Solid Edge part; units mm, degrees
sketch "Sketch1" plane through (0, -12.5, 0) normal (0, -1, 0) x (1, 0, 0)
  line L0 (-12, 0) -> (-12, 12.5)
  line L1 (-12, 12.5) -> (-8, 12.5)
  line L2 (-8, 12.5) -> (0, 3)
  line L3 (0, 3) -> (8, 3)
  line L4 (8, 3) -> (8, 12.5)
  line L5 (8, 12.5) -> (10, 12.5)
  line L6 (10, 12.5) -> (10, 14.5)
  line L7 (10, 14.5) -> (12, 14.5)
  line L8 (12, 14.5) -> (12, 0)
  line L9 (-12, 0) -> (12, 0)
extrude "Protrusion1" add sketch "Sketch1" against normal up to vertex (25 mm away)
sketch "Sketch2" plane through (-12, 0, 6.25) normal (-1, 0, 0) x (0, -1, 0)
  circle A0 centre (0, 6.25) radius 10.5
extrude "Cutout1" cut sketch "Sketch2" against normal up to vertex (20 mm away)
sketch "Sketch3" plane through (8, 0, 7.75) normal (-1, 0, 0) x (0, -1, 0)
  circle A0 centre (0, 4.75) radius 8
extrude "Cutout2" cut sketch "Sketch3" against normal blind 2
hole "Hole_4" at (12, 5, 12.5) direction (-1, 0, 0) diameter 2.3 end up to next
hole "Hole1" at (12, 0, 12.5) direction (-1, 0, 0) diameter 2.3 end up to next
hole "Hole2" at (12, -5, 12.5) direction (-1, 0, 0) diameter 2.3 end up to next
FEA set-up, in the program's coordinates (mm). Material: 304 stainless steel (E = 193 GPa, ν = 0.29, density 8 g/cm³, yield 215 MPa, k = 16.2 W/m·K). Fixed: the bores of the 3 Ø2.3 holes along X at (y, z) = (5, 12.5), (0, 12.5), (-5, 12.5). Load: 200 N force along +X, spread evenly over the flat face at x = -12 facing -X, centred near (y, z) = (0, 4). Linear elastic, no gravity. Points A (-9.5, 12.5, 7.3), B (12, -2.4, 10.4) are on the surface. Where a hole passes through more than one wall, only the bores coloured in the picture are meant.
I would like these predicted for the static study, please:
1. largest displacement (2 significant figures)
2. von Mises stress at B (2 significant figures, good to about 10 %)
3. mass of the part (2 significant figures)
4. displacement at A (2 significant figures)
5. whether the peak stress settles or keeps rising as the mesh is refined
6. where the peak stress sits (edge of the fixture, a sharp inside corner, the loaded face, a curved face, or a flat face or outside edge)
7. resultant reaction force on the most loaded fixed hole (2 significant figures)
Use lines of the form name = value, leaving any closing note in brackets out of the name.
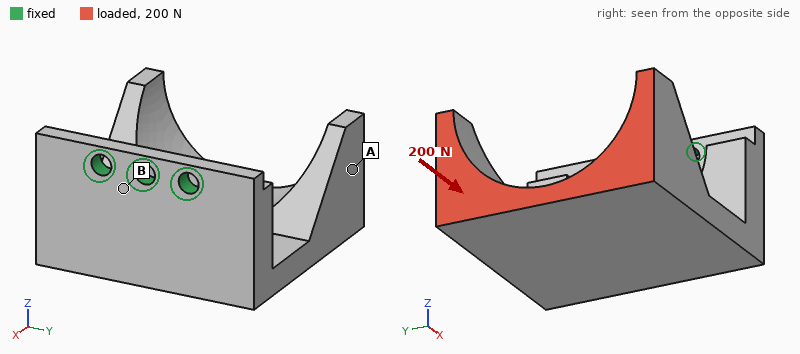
largest displacement = 28 µm
von Mises stress at B = 66 MPa
mass of the part = 25 g
displacement at A = 23 µm
whether the peak stress settles or keeps rising as the mesh is refined = keeps rising
where the peak stress sits = edge of the fixture
resultant reaction force on the most loaded fixed hole = 75 N
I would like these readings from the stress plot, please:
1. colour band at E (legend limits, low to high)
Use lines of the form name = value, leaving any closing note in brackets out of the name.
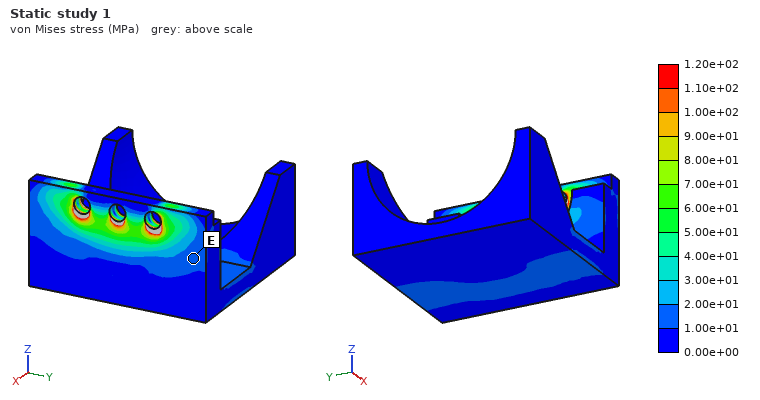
colour band at E = 1.00e+01 to 2.00e+01 MPa
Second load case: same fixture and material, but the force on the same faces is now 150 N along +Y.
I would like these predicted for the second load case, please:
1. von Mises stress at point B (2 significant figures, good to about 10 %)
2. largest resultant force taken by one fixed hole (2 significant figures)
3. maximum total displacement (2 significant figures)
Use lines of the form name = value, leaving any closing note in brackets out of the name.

von Mises stress at point B = 44 MPa
largest resultant force taken by one fixed hole = 260 N
maximum total displacement = 62 µm
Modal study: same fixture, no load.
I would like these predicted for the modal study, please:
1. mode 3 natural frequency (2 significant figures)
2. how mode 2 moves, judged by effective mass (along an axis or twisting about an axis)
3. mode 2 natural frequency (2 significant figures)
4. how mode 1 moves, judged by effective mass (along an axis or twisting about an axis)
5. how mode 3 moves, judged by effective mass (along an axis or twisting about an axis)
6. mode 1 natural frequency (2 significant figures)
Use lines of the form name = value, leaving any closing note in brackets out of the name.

mode 3 natural frequency = 5900 Hz
how mode 2 moves, judged by effective mass = along Y
mode 2 natural frequency = 2800 Hz
how mode 1 moves, judged by effective mass = along Z
how mode 3 moves, judged by effective mass = along X
mode 1 natural frequency = 1800 Hz
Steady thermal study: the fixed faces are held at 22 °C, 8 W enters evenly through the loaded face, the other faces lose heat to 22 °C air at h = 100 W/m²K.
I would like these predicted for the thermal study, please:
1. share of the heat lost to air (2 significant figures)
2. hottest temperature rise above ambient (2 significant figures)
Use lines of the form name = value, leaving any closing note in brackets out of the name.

share of the heat lost to air = 85 %
hottest temperature rise above ambient = 69 K
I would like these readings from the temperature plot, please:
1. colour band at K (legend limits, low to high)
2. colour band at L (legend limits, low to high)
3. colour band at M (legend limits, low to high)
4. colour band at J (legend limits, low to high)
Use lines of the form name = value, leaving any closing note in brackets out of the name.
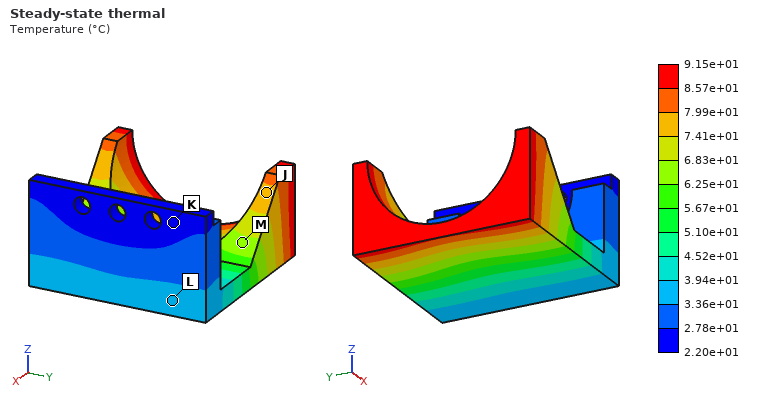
colour band at K = 2.20e+01 to 2.78e+01 °C
colour band at L = 3.36e+01 to 3.94e+01 °C
colour band at M = 6.25e+01 to 6.83e+01 °C
colour band at J = 7.41e+01 to 7.99e+01 °C
